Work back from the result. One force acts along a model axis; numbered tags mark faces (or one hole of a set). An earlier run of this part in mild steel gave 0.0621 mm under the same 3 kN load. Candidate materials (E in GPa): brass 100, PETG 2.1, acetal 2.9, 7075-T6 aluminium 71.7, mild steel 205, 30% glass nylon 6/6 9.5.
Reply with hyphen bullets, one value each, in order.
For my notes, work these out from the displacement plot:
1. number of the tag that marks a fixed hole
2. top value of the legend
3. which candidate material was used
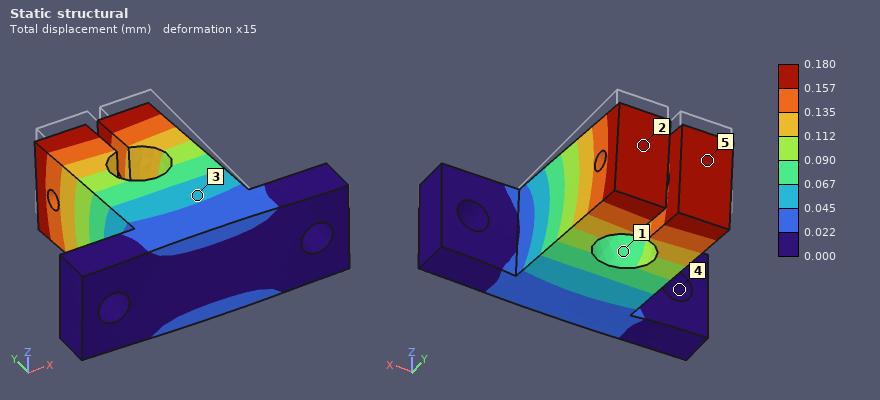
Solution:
- 4
- 0.180 mm
- 7075-T6 aluminium
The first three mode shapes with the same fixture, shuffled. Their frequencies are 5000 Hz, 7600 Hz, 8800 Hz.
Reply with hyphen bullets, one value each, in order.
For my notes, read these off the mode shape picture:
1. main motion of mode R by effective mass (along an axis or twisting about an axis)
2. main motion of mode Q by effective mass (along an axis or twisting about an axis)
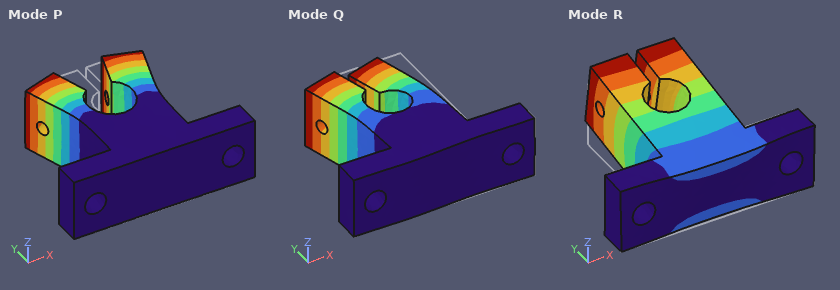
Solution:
- along Z
- along X
